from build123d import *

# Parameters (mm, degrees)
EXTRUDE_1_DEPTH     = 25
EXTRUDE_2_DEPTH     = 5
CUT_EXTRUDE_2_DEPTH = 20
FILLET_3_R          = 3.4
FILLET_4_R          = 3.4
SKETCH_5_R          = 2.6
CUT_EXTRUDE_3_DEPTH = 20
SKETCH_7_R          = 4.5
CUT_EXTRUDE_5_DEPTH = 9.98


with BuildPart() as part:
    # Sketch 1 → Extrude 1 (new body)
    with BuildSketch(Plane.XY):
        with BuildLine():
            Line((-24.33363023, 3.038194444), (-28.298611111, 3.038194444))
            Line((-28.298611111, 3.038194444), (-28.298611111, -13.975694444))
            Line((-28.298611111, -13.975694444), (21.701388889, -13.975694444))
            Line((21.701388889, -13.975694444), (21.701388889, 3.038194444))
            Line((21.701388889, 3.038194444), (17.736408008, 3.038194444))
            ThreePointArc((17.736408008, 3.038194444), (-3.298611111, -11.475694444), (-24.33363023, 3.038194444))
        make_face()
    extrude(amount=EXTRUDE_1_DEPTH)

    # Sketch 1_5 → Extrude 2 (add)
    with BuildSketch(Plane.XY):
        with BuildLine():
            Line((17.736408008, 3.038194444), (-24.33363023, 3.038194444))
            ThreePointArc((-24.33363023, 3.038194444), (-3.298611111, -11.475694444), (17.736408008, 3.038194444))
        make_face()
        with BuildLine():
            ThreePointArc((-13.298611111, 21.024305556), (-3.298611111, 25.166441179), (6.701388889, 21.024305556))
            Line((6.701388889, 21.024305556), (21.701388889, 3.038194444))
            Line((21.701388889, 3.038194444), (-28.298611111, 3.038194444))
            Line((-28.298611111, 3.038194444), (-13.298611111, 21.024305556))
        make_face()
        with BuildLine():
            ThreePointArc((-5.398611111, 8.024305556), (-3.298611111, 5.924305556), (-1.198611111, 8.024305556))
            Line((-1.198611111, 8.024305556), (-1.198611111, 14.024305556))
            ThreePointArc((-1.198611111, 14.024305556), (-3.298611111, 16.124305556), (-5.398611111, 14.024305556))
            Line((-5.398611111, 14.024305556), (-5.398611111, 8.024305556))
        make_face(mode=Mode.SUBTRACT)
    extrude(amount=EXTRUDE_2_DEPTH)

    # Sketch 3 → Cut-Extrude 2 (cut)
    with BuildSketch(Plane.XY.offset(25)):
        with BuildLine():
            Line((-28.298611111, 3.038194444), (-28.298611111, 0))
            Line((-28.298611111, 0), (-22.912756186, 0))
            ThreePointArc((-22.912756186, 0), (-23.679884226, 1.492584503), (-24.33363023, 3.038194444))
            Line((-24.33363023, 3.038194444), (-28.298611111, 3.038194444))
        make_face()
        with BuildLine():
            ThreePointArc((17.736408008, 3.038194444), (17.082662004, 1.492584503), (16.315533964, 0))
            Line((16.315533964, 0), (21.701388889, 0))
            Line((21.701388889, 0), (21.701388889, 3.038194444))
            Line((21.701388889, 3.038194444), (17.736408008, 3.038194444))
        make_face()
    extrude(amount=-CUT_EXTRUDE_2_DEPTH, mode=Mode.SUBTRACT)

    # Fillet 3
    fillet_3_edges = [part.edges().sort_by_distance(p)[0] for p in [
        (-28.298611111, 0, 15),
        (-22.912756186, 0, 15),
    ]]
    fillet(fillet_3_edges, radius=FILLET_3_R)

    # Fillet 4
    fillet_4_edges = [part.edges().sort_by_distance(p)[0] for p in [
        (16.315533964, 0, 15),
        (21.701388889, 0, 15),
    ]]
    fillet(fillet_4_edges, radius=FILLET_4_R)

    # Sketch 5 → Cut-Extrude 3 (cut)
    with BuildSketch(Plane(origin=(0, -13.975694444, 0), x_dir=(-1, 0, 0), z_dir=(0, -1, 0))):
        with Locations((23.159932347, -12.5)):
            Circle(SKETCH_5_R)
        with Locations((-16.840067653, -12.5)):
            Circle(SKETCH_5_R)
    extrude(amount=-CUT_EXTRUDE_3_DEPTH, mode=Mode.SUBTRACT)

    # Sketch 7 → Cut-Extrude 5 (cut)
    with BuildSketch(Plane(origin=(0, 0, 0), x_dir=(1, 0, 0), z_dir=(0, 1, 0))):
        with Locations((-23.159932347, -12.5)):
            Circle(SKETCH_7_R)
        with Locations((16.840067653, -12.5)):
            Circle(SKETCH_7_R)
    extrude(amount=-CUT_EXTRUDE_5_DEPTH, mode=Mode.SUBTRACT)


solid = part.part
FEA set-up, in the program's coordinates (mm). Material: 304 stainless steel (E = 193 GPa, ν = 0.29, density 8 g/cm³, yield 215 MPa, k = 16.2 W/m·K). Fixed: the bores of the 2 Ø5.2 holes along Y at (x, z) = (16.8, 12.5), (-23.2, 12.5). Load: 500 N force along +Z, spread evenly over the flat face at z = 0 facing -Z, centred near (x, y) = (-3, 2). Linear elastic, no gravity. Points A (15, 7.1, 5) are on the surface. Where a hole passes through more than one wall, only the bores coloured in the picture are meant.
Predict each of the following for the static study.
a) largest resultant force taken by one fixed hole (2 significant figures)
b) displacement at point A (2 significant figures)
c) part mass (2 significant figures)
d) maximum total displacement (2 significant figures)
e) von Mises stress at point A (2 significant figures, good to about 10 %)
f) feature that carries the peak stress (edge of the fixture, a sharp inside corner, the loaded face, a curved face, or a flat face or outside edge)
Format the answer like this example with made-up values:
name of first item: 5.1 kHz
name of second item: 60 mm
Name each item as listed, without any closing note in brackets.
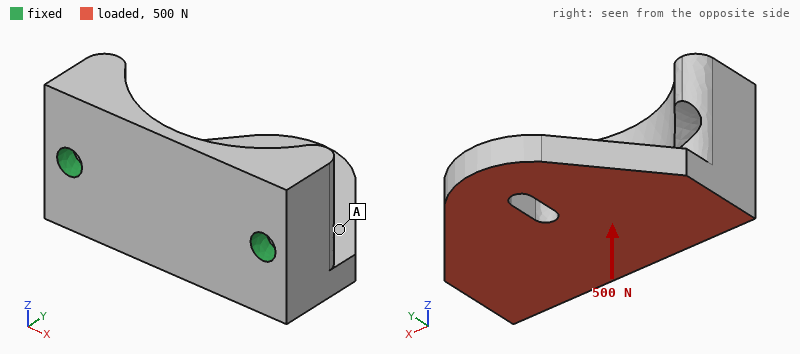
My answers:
largest resultant force taken by one fixed hole: 250 N
displacement at point A: 12 µm
part mass: 110 g
maximum total displacement: 32 µm
von Mises stress at point A: 9.0 MPa
feature that carries the peak stress: a curved face
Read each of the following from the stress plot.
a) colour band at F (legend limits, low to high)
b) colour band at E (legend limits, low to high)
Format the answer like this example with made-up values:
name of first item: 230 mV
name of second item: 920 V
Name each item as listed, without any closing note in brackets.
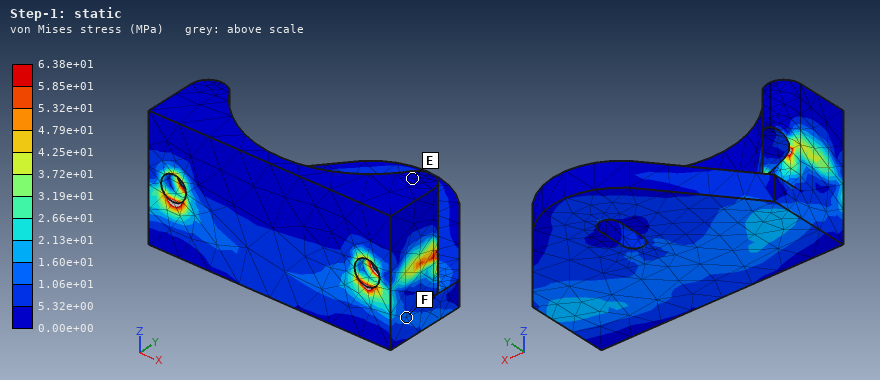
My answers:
colour band at F: 1.06e+01 to 1.60e+01 MPa
colour band at E: 0.00e+00 to 5.32e+00 MPa
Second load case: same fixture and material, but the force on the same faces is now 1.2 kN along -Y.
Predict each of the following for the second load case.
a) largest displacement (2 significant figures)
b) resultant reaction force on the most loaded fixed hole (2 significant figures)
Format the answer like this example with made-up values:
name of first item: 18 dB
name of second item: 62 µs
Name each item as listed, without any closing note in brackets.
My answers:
largest displacement: 39 µm
resultant reaction force on the most loaded fixed hole: 610 N
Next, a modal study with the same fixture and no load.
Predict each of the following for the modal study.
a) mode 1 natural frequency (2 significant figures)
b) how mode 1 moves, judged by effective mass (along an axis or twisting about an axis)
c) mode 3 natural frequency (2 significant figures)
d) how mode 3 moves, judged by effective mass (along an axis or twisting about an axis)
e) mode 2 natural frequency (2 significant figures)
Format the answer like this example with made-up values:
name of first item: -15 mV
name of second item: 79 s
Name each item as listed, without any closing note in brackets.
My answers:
mode 1 natural frequency: 3400 Hz
how mode 1 moves, judged by effective mass: along Z
mode 3 natural frequency: 10 kHz
how mode 3 moves, judged by effective mass: along Y
mode 2 natural frequency: 8500 Hz
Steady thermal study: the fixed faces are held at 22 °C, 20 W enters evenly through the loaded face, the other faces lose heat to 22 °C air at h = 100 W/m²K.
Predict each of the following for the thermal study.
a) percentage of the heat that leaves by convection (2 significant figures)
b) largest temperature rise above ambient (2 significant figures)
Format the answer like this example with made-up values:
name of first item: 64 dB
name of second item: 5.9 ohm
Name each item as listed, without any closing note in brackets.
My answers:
percentage of the heat that leaves by convection: 59 %
largest temperature rise above ambient: 55 K
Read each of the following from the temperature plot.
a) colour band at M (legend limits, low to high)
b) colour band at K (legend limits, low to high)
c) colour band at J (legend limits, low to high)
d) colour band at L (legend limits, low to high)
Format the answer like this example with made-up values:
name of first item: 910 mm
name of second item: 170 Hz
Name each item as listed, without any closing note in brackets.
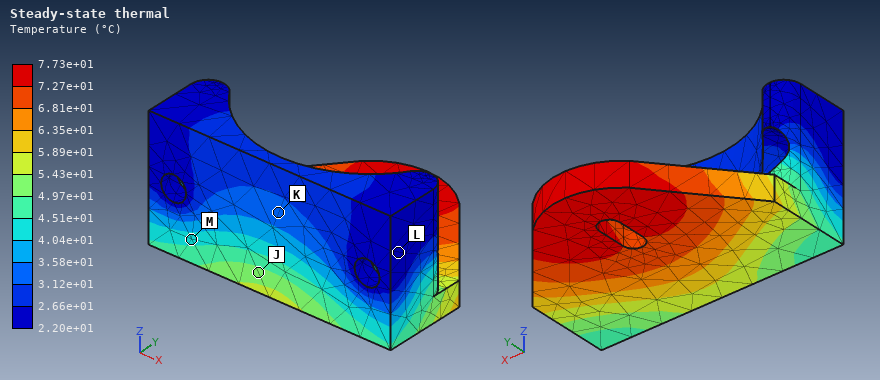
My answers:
colour band at M: 4.04e+01 to 4.51e+01 °C
colour band at K: 3.12e+01 to 3.58e+01 °C
colour band at J: 4.97e+01 to 5.43e+01 °C
colour band at L: 2.20e+01 to 2.66e+01 °C
